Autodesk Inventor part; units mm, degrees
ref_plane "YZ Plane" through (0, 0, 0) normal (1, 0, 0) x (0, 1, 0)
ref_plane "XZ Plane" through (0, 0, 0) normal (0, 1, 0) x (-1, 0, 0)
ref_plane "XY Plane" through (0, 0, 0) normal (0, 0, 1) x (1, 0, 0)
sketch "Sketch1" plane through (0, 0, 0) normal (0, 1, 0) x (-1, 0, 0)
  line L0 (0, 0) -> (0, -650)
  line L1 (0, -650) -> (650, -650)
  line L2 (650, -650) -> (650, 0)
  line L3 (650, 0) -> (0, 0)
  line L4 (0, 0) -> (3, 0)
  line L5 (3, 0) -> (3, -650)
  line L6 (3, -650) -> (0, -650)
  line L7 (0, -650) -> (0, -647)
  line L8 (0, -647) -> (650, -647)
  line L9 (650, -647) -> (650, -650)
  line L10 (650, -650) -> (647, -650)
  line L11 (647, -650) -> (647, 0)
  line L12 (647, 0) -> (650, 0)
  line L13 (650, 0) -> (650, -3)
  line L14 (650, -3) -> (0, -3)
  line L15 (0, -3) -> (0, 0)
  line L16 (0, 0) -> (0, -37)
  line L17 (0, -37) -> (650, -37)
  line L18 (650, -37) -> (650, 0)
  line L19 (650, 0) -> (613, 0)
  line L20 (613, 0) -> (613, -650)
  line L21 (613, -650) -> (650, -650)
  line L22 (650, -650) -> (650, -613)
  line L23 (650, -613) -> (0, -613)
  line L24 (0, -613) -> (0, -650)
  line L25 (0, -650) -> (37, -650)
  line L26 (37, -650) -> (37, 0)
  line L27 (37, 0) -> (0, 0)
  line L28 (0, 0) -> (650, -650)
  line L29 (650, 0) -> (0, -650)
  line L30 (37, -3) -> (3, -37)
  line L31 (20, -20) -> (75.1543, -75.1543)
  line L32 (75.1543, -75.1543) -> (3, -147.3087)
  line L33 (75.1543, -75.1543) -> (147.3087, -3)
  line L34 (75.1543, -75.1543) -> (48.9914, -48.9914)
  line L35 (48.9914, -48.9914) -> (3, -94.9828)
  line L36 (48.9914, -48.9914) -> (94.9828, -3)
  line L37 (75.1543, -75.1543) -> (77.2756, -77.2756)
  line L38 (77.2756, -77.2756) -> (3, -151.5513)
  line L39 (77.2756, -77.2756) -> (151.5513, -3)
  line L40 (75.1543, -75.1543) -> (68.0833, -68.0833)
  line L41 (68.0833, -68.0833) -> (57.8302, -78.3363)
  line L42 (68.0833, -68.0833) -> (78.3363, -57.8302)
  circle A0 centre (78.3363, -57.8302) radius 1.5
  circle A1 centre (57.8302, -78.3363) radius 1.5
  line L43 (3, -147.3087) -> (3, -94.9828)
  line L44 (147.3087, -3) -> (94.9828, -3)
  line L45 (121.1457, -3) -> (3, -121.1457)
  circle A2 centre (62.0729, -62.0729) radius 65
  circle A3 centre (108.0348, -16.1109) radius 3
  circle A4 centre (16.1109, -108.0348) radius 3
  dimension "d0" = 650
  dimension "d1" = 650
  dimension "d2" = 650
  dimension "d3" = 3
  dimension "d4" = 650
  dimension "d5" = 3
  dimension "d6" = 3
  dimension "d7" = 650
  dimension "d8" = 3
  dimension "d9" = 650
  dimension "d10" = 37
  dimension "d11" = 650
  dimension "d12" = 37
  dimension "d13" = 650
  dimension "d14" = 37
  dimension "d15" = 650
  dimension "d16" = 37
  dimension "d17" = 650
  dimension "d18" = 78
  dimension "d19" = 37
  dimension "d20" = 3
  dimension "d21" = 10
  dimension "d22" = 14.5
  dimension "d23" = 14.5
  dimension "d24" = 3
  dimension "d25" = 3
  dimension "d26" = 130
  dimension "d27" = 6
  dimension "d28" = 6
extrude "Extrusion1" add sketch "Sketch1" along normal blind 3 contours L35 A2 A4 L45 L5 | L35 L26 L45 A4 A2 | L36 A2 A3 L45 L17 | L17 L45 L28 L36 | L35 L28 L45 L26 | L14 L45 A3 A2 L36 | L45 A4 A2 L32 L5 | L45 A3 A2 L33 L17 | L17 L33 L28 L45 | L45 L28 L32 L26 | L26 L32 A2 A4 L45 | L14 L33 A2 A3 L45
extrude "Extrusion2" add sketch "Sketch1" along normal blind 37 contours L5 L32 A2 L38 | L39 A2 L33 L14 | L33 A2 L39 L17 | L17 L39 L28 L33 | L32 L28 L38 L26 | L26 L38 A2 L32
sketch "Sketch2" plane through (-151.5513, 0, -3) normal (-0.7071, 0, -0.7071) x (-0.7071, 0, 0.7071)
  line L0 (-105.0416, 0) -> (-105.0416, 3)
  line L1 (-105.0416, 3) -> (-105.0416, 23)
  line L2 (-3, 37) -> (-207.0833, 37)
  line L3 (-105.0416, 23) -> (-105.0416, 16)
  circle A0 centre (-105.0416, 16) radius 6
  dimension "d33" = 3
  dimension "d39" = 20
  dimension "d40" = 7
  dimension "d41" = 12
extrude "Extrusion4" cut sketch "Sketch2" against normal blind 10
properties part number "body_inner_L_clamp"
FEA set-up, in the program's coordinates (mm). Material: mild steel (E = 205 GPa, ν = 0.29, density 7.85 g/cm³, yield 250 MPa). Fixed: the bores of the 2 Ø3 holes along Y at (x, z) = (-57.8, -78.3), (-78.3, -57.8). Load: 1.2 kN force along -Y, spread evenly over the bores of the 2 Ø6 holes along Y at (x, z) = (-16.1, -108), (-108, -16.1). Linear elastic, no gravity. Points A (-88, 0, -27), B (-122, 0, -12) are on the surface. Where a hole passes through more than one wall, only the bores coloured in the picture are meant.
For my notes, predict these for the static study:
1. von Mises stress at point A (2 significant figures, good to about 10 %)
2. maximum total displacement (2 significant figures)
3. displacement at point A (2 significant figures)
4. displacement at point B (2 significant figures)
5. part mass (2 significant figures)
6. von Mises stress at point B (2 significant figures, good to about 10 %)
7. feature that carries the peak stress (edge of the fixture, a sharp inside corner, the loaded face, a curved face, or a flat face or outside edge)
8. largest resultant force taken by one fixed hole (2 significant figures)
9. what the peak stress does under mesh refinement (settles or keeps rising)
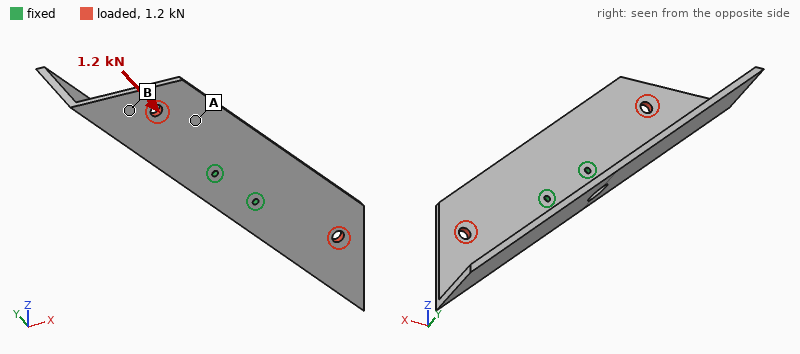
74 MPa
0.43 mm
0.18 mm
0.17 mm
320 g
21 MPa
edge of the fixture
810 N
keeps rising
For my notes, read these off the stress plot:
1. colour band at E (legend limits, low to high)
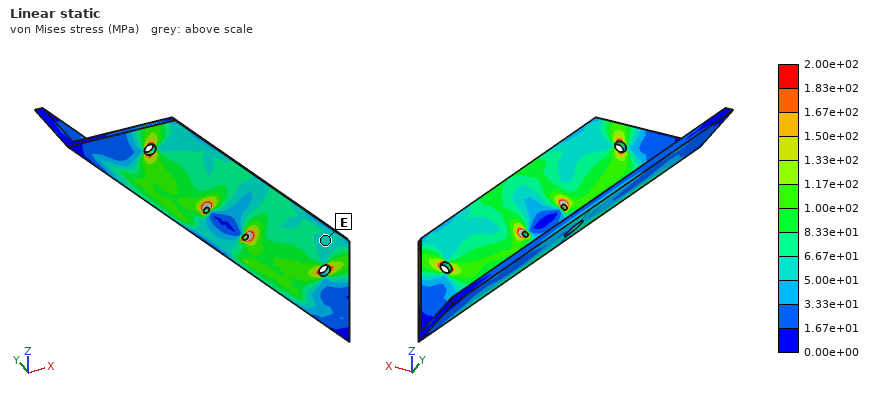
5.00e+01 to 6.67e+01 MPa
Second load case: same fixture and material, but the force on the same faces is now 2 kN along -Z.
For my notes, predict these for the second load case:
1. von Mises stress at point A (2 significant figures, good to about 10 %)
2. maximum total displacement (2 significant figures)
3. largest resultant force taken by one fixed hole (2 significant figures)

11 MPa
42 µm
1.2 kN
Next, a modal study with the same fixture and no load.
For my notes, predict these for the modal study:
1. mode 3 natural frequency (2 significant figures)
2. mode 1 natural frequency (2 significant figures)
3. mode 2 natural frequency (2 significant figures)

870 Hz
660 Hz
710 Hz
